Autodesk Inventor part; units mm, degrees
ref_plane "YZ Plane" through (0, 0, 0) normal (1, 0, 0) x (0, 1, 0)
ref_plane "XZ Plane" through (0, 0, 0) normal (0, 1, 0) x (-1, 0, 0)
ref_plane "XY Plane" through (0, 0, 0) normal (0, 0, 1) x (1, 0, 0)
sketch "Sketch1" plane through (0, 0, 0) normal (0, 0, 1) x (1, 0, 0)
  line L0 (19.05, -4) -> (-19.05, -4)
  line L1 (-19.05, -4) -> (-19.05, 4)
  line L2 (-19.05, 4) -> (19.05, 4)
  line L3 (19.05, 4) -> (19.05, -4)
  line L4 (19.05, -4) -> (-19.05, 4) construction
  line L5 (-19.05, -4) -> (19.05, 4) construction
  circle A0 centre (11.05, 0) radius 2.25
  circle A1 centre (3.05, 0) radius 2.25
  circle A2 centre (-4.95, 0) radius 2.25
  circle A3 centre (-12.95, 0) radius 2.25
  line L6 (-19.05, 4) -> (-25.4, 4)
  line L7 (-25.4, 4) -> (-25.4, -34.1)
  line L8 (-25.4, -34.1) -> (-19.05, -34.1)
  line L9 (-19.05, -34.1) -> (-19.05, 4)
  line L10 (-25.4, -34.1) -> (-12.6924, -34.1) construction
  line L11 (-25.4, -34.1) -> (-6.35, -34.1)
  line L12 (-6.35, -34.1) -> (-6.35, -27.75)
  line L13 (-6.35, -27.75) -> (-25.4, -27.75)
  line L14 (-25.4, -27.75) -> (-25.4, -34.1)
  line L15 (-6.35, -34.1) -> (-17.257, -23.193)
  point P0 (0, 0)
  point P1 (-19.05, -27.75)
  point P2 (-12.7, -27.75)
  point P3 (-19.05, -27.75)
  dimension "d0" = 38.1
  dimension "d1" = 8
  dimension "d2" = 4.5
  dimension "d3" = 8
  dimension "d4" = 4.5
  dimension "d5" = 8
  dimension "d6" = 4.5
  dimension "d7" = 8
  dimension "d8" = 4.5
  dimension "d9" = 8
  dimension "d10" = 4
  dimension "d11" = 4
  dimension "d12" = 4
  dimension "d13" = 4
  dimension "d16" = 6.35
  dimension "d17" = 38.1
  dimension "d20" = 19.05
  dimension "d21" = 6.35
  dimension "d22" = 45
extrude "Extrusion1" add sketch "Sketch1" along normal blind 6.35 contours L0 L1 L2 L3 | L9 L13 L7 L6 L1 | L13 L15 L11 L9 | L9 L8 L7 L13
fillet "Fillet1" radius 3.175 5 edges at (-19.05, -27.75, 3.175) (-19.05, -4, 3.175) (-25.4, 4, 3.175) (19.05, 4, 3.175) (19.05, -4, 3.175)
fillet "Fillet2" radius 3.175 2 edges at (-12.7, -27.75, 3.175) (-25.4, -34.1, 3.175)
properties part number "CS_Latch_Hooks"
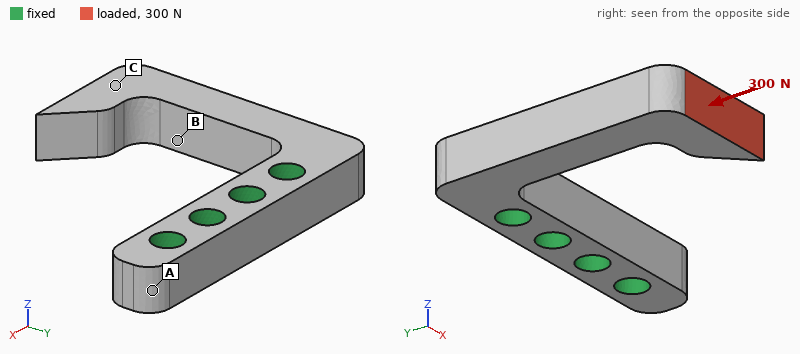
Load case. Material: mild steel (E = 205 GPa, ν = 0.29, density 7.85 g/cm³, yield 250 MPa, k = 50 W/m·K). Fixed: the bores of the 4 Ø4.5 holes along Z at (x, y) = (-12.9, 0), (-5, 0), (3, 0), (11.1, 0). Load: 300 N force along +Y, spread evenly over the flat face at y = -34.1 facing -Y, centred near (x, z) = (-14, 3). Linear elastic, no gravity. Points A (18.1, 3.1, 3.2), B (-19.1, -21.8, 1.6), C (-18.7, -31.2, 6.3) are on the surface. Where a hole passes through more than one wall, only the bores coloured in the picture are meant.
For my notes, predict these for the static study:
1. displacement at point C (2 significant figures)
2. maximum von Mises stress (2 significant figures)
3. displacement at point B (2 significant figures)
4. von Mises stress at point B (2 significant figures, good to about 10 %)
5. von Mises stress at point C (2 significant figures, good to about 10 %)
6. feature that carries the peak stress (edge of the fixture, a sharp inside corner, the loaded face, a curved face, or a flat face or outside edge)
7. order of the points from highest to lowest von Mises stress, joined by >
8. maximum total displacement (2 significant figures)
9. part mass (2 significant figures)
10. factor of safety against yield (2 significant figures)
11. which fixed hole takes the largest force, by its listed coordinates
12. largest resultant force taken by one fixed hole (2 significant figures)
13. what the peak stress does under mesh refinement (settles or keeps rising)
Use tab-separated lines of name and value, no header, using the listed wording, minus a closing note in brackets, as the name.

displacement at point C	37 µm
maximum von Mises stress	84 MPa
displacement at point B	17 µm
von Mises stress at point B	63 MPa
von Mises stress at point C	14 MPa
feature that carries the peak stress	a curved face
order of the points from highest to lowest von Mises stress, joined by >	B > C > A
maximum total displacement	59 µm
part mass	27 g
factor of safety against yield	3.0
which fixed hole takes the largest force, by its listed coordinates	(-12.9, 0)
largest resultant force taken by one fixed hole	300 N
what the peak stress does under mesh refinement	settles
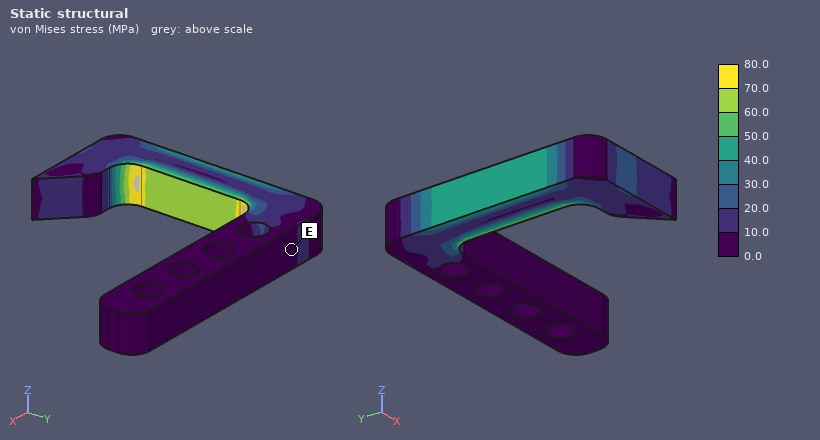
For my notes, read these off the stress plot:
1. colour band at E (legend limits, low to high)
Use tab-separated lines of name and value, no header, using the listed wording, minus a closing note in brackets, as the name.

colour band at E	0.0 to 10.0 MPa
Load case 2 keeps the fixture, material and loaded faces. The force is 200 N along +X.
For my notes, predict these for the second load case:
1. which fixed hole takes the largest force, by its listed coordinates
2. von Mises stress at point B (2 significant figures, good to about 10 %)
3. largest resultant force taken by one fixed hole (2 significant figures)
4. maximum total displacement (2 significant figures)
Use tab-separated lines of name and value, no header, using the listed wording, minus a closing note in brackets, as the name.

which fixed hole takes the largest force, by its listed coordinates	(-12.9, 0)
von Mises stress at point B	58 MPa
largest resultant force taken by one fixed hole	220 N
maximum total displacement	0.12 mm
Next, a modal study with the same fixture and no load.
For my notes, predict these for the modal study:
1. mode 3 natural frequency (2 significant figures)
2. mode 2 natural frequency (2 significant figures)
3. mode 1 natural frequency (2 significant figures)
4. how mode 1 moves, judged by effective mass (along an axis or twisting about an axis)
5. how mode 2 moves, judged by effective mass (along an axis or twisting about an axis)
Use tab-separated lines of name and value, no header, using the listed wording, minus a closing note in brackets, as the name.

mode 3 natural frequency	9200 Hz
mode 2 natural frequency	3000 Hz
mode 1 natural frequency	2700 Hz
how mode 1 moves, judged by effective mass	along Z
how mode 2 moves, judged by effective mass	along X
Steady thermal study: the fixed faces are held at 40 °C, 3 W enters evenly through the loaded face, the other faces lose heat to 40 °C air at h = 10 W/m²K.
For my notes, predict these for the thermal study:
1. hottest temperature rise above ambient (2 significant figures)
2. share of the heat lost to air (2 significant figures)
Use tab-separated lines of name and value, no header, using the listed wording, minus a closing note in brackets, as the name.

hottest temperature rise above ambient	55 K
share of the heat lost to air	11 %
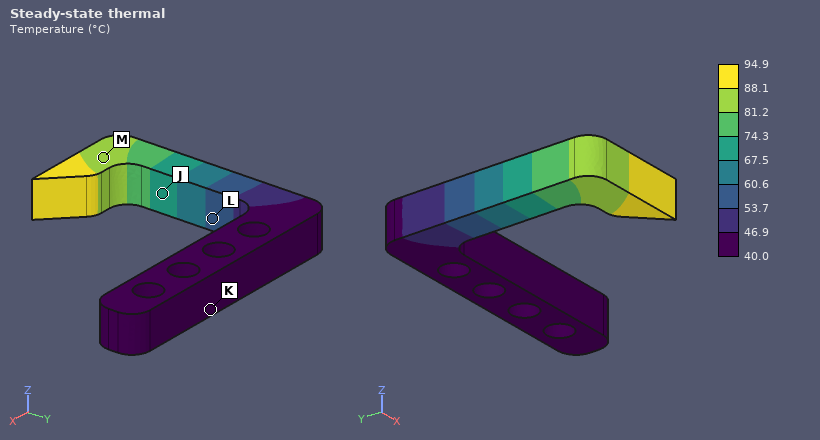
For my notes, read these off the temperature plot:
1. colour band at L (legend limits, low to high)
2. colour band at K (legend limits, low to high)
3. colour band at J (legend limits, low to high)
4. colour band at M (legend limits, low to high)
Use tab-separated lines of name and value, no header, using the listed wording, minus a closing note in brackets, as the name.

colour band at L	53.7 to 60.6 °C
colour band at K	40.0 to 46.9 °C
colour band at J	67.5 to 74.3 °C
colour band at M	81.2 to 88.1 °C
